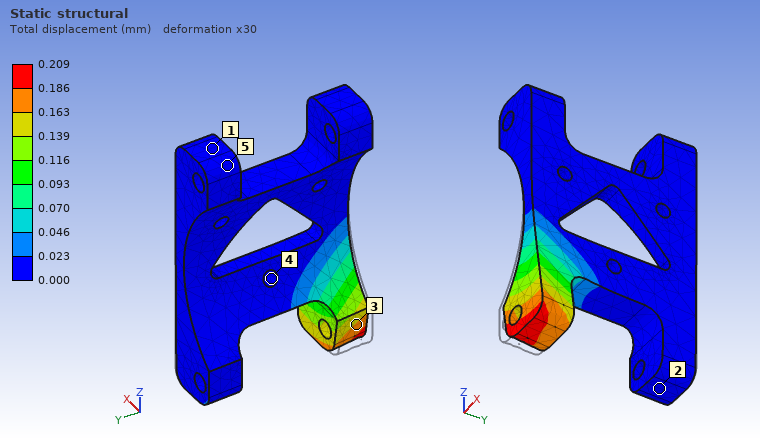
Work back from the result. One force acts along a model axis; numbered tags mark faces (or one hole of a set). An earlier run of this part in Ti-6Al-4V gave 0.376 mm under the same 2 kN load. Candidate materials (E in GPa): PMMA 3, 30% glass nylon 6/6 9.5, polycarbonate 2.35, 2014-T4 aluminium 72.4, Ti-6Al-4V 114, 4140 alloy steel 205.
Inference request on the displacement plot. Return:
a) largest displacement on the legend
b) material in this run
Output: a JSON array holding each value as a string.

["0.209 mm", "4140 alloy steel"]
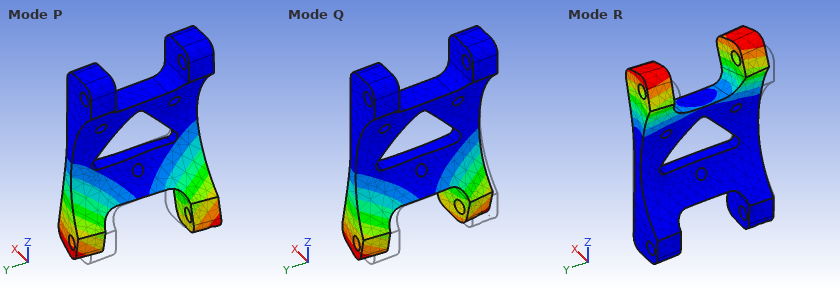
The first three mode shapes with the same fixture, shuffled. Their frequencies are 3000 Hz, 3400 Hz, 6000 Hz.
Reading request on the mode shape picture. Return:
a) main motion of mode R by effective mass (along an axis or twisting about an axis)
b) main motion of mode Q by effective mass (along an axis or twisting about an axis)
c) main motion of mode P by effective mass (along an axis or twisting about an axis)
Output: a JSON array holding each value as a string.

["along X", "along X", "twisting about Z"]
